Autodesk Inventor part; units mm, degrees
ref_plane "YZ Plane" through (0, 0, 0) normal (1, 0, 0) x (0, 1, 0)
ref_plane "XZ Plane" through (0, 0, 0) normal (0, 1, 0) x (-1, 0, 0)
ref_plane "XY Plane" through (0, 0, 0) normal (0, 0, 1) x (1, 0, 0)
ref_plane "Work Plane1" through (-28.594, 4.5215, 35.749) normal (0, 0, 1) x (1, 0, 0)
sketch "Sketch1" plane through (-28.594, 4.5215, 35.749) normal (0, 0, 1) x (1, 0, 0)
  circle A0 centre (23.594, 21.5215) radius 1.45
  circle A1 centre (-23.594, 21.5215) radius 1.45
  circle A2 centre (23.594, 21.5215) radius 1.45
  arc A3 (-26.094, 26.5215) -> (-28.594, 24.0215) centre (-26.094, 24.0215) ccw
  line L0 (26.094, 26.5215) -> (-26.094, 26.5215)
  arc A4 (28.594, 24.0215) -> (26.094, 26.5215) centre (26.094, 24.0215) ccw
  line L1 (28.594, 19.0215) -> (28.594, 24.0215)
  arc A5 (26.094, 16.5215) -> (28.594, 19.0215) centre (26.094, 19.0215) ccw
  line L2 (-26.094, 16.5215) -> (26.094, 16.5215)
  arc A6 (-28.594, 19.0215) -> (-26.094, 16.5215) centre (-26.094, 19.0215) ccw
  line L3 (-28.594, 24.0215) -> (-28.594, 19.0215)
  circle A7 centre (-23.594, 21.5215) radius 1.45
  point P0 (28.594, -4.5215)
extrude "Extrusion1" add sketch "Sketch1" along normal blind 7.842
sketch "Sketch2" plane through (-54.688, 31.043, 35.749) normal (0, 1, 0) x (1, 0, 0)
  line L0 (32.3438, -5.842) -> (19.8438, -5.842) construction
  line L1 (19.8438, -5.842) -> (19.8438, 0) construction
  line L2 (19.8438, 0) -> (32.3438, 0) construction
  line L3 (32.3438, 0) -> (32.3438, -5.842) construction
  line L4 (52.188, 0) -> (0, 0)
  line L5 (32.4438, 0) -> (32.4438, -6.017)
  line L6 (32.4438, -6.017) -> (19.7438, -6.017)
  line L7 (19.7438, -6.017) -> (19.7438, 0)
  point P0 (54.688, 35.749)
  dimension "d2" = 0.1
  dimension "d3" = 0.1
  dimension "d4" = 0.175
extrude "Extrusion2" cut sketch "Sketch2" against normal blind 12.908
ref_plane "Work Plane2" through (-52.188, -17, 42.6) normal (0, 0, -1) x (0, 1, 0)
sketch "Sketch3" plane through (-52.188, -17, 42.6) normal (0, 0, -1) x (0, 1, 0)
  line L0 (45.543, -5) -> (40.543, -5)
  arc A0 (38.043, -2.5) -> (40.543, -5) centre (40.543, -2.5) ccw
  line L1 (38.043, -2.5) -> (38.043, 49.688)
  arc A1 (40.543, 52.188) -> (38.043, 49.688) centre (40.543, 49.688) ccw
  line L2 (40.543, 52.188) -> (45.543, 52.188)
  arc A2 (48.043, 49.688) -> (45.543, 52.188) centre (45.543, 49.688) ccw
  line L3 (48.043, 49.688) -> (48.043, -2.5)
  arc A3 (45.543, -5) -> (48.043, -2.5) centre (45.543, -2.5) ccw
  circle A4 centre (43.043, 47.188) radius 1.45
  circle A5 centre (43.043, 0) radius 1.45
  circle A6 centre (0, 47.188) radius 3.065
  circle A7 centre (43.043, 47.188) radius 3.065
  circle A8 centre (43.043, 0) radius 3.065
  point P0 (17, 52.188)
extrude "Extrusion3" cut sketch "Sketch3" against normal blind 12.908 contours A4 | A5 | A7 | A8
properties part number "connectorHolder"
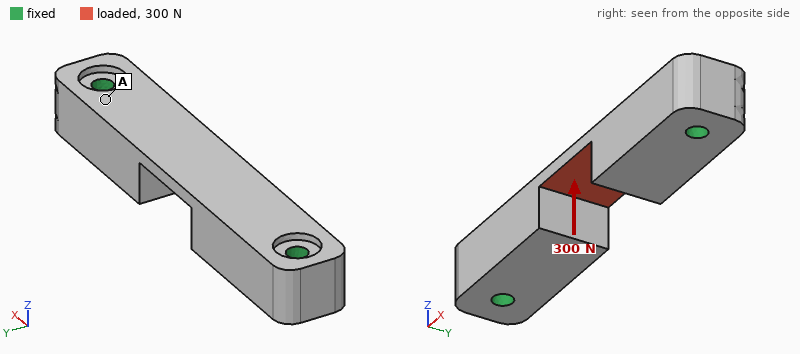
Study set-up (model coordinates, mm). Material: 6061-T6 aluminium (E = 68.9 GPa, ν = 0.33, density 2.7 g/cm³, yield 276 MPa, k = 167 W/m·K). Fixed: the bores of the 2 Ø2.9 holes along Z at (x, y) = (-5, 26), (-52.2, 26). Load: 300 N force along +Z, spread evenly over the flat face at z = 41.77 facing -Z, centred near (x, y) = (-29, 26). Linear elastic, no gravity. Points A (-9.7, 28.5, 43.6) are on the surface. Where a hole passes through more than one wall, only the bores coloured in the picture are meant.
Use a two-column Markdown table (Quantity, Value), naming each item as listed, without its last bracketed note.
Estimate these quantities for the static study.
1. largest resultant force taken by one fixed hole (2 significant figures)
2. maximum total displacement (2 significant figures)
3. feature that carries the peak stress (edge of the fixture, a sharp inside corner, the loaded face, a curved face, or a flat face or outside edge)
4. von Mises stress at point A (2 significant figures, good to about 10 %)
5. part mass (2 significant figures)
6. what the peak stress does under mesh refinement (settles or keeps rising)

| Quantity | Value |
|---|---|
| largest resultant force taken by one fixed hole | 280 N |
| maximum total displacement | 20 µm |
| feature that carries the peak stress | edge of the fixture |
| von Mises stress at point A | 9.2 MPa |
| part mass | 9.5 g |
| what the peak stress does under mesh refinement | keeps rising |
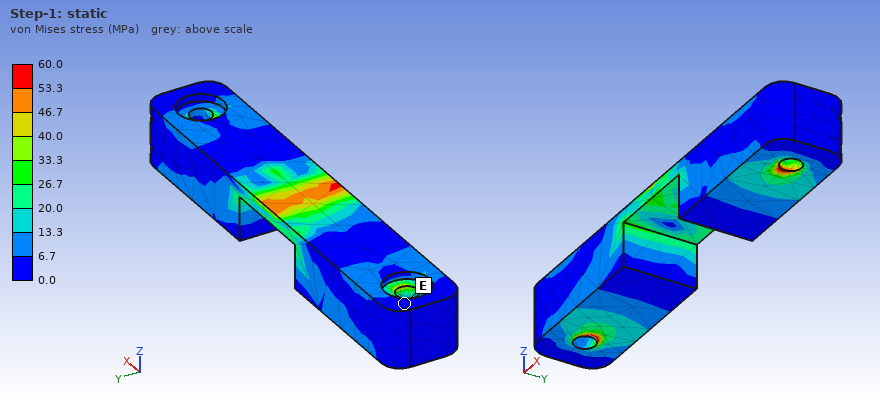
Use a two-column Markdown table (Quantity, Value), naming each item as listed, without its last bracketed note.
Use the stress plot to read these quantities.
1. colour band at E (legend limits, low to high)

| Quantity | Value |
|---|---|
| colour band at E | 0.0 to 6.7 MPa |
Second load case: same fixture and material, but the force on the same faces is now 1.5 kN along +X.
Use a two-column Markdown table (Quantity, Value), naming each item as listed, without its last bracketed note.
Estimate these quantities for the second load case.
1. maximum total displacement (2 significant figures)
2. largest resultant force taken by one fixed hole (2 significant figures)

| Quantity | Value |
|---|---|
| maximum total displacement | 16 µm |
| largest resultant force taken by one fixed hole | 750 N |
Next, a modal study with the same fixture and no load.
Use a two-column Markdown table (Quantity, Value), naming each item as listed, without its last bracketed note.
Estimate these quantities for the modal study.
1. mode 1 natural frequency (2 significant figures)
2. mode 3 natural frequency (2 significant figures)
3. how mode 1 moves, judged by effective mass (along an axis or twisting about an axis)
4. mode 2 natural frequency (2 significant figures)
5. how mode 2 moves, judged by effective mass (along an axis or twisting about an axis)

| Quantity | Value |
|---|---|
| mode 1 natural frequency | 15 kHz |
| mode 3 natural frequency | 19 kHz |
| how mode 1 moves, judged by effective mass | along Y |
| mode 2 natural frequency | 17 kHz |
| how mode 2 moves, judged by effective mass | along Z |
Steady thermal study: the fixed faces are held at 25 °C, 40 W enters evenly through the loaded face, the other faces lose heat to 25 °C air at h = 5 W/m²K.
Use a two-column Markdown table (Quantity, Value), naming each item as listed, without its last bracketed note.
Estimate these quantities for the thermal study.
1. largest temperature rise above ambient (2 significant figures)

| Quantity | Value |
|---|---|
| largest temperature rise above ambient | 56 K |
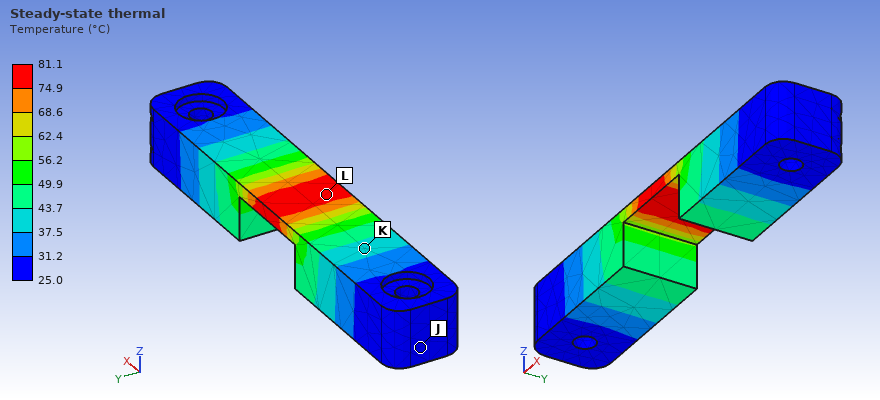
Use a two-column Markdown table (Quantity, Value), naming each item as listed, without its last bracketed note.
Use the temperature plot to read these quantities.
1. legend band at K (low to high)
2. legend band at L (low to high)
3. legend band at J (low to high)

| Quantity | Value |
|---|---|
| legend band at K | 37.5 to 43.7 °C |
| legend band at L | 74.9 to 81.1 °C |
| legend band at J | 25.0 to 31.2 °C |
